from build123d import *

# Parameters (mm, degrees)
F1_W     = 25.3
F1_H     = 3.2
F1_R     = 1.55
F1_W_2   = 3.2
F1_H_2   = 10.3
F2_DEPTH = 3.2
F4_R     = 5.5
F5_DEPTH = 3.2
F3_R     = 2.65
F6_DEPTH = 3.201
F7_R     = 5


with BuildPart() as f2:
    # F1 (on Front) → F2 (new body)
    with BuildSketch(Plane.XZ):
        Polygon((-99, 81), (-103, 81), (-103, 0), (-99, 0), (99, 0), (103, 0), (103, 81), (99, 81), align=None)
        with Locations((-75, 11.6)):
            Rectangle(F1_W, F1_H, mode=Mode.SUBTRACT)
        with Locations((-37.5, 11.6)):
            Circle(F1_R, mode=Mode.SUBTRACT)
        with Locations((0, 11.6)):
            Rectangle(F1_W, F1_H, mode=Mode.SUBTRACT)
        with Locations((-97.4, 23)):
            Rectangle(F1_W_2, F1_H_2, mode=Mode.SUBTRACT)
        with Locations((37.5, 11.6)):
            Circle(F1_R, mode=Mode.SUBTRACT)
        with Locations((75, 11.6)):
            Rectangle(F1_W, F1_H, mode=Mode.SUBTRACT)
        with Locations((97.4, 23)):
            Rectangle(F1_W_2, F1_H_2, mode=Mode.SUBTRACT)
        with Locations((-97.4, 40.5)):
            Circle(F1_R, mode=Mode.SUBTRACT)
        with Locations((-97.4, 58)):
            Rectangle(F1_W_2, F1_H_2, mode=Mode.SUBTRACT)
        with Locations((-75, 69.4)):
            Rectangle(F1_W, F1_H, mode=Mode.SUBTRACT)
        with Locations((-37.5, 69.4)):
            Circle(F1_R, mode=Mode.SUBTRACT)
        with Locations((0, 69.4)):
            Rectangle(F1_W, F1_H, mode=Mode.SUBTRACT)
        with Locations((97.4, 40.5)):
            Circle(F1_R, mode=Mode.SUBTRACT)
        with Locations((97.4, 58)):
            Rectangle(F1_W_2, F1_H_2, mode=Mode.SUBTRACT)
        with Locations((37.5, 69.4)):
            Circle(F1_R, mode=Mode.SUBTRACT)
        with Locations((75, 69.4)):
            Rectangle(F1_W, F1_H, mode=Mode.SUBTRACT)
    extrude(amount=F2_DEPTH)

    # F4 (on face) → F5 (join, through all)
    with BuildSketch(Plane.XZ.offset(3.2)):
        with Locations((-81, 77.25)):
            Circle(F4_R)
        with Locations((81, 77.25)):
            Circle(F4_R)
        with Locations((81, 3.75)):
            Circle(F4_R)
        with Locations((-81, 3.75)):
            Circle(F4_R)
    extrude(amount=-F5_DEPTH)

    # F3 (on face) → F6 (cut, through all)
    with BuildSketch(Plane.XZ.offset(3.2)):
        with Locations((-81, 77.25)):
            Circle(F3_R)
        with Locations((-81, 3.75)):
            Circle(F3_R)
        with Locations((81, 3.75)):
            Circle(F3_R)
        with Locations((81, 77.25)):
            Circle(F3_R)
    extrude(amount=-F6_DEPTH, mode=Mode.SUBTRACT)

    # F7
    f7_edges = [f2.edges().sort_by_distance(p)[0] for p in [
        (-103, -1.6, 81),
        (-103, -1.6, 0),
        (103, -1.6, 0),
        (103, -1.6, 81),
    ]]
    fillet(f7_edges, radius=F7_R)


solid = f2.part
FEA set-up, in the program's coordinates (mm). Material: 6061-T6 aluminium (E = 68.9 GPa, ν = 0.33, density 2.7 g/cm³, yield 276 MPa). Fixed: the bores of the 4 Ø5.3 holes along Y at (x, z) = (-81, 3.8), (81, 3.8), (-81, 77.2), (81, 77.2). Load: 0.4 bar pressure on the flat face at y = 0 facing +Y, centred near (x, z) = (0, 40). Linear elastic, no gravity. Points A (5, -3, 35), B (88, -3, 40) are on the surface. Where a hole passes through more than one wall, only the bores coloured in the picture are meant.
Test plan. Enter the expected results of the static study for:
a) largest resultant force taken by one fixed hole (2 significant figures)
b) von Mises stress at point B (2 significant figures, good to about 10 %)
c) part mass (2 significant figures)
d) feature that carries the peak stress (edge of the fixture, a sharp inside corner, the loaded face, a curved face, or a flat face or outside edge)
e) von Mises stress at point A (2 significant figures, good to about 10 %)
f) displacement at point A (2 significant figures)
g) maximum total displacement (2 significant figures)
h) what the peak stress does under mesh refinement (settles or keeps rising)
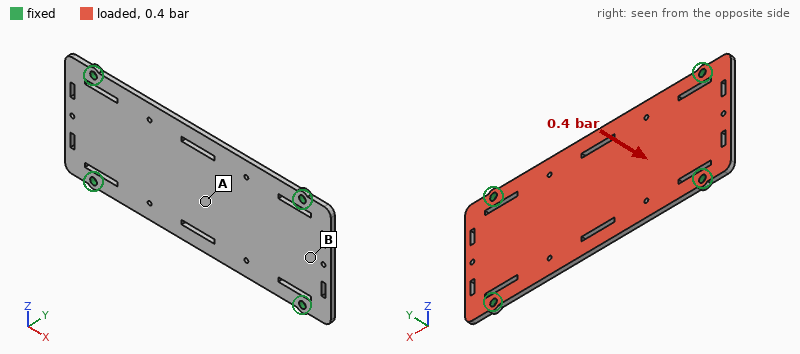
160 N
13 MPa
140 g
edge of the fixture
28 MPa
0.55 mm
0.57 mm
keeps rising
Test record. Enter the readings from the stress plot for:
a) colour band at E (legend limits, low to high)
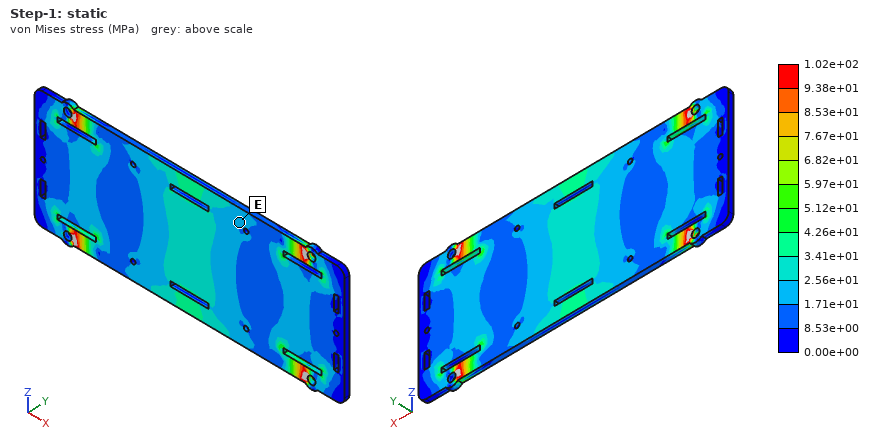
1.71e+01 to 2.56e+01 MPa
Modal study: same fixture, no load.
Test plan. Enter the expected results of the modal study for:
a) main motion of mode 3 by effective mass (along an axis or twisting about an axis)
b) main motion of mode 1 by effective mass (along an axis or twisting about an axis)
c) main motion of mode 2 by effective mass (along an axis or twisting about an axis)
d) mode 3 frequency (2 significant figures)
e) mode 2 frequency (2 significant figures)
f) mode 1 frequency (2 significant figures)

twisting about Z
along Y
twisting about X
1400 Hz
1000 Hz
520 Hz
